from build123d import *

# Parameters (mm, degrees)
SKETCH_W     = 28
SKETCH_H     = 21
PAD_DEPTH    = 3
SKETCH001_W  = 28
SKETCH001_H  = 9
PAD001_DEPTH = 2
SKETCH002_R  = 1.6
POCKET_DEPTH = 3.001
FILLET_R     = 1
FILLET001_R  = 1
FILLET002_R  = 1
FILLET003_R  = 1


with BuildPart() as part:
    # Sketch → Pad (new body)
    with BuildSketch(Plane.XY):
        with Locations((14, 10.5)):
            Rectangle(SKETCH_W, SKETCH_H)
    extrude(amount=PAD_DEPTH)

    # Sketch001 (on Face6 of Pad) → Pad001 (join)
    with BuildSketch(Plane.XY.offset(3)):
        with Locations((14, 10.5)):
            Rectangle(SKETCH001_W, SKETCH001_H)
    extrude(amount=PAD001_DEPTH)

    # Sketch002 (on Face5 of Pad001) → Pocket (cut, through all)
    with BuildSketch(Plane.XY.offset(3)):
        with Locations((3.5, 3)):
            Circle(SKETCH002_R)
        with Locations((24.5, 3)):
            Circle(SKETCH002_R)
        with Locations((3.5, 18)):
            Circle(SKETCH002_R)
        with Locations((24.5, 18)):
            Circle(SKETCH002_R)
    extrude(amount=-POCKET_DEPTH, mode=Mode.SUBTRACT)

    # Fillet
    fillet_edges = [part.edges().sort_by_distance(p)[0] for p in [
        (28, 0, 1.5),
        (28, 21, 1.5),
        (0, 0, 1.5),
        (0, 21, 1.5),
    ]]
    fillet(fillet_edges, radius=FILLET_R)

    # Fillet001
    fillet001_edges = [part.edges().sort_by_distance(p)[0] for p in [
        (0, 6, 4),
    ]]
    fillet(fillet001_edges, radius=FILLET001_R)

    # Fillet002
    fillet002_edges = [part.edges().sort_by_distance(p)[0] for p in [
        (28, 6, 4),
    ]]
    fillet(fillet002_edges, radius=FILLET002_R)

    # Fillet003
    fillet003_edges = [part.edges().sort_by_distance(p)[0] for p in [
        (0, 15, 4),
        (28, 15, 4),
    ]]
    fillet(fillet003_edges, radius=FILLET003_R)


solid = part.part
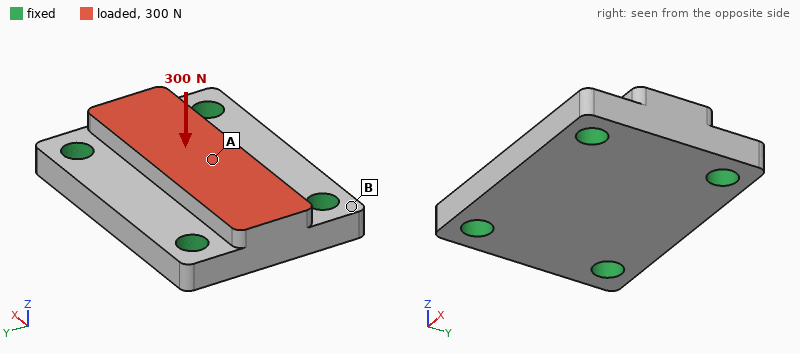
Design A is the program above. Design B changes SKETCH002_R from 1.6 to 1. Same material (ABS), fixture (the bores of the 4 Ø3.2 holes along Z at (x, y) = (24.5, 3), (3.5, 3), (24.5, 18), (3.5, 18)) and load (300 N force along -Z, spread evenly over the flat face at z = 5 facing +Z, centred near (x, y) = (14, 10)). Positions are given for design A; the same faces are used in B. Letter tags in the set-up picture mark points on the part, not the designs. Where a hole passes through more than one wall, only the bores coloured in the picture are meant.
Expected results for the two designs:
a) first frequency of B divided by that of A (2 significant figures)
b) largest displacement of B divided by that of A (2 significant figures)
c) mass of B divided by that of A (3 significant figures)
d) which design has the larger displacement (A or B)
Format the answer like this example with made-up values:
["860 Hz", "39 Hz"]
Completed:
["0.87", "1.3", "1.03", "B"]
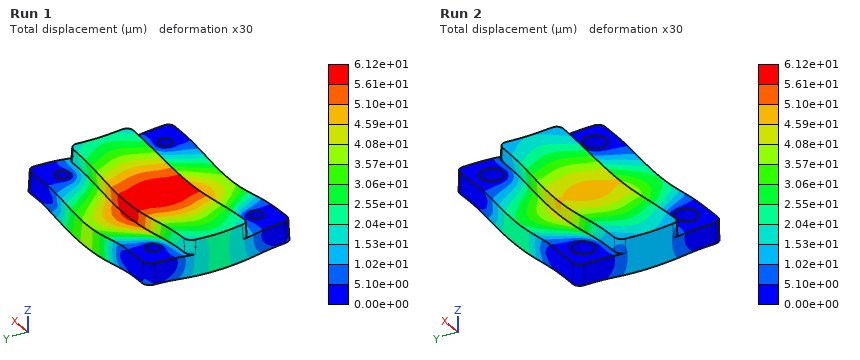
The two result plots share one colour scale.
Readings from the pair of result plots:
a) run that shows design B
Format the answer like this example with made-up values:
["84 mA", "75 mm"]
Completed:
["Run 1"]
